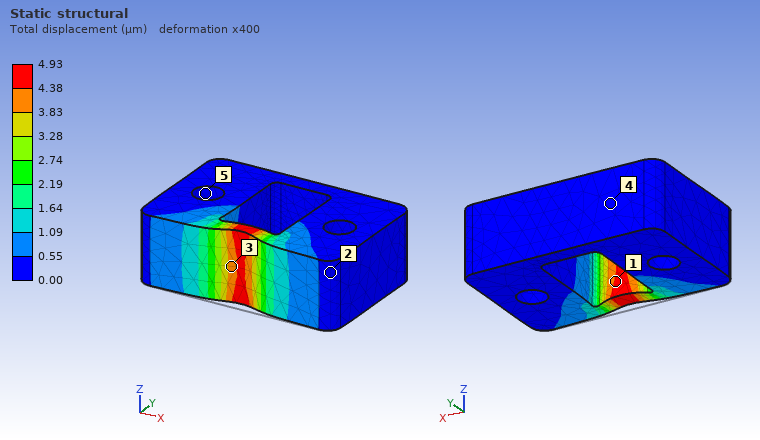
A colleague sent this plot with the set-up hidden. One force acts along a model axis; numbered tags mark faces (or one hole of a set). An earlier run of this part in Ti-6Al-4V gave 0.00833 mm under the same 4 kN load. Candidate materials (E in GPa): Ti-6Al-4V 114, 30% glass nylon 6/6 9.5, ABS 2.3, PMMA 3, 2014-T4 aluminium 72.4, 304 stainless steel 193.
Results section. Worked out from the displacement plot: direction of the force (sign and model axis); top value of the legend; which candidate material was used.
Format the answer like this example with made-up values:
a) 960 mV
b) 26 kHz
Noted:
a) +Y
b) 4.93 µm
c) 304 stainless steel
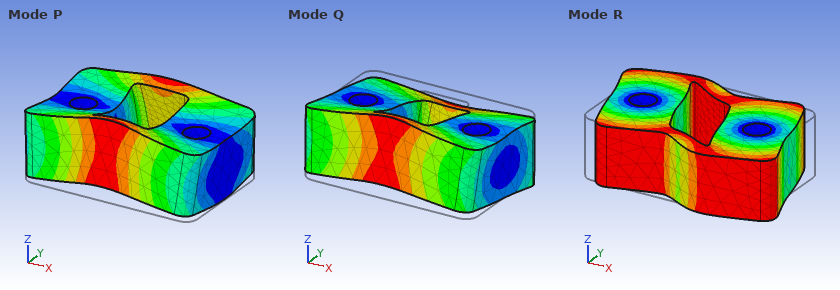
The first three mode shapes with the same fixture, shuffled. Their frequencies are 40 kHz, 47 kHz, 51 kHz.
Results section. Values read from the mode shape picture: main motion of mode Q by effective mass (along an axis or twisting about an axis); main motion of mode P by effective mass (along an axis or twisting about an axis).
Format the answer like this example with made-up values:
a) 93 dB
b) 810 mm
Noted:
a) twisting about X
b) along Z
